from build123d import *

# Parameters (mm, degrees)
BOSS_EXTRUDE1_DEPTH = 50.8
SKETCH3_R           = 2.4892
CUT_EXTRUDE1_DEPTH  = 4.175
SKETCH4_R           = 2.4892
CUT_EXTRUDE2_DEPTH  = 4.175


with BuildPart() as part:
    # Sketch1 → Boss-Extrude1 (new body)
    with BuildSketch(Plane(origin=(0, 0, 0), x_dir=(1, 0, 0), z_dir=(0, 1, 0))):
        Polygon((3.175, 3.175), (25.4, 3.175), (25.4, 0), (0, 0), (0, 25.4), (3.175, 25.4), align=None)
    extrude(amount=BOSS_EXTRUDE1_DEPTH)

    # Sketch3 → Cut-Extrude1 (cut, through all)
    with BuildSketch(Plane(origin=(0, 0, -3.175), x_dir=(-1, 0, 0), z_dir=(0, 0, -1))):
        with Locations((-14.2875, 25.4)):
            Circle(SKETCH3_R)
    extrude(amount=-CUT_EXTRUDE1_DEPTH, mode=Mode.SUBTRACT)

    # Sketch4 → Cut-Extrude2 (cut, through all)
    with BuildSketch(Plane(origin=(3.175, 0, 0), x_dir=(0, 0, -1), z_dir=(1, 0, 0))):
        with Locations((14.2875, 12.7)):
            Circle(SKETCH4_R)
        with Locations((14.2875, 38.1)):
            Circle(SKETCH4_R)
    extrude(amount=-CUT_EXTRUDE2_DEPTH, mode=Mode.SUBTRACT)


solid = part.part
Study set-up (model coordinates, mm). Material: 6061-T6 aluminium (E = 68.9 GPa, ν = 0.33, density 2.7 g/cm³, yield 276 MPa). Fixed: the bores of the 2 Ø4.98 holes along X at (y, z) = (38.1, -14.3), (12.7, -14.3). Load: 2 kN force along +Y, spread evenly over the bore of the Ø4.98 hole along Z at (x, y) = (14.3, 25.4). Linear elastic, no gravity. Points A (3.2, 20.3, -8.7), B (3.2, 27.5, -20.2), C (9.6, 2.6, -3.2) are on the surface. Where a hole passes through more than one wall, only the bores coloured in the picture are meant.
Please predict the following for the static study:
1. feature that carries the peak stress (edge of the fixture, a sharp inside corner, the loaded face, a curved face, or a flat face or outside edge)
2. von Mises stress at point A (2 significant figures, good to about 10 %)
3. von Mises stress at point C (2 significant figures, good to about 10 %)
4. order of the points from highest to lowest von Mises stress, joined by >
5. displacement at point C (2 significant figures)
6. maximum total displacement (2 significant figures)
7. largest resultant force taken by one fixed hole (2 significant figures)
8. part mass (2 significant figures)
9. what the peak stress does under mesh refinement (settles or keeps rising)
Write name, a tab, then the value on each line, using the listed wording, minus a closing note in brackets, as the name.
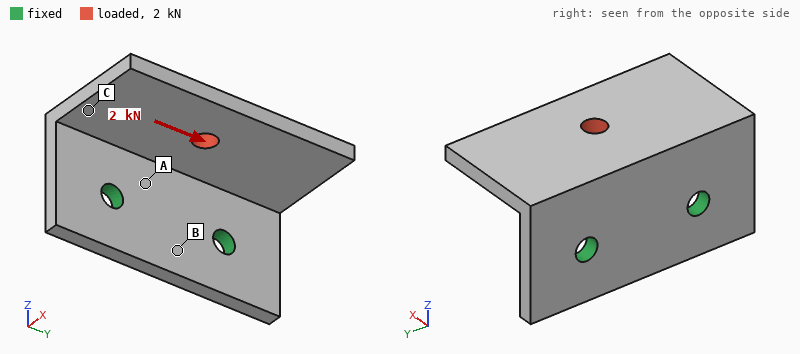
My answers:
feature that carries the peak stress	edge of the fixture
von Mises stress at point A	93 MPa
von Mises stress at point C	51 MPa
order of the points from highest to lowest von Mises stress, joined by >	A > C > B
displacement at point C	0.13 mm
maximum total displacement	0.22 mm
largest resultant force taken by one fixed hole	1.5 kN
part mass	20 g
what the peak stress does under mesh refinement	keeps rising
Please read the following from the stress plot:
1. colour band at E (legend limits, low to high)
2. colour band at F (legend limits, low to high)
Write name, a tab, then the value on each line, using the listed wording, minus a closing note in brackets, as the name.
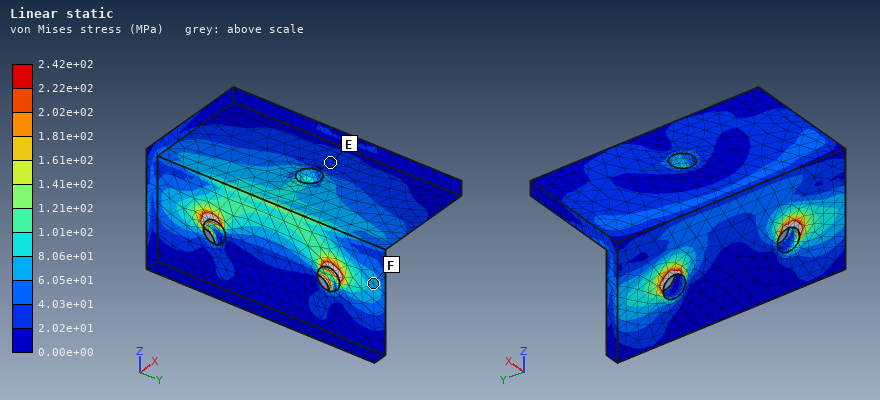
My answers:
colour band at E	2.02e+01 to 4.03e+01 MPa
colour band at F	6.05e+01 to 8.06e+01 MPa
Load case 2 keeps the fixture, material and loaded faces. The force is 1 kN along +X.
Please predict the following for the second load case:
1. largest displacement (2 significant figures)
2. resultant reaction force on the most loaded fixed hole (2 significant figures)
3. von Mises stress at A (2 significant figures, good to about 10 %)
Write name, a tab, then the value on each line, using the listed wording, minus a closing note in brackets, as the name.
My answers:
largest displacement	0.21 mm
resultant reaction force on the most loaded fixed hole	500 N
von Mises stress at A	65 MPa
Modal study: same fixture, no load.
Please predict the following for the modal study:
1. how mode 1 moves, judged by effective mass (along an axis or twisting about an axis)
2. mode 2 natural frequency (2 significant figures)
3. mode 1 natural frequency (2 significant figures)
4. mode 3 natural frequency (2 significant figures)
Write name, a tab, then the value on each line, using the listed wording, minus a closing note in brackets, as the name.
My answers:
how mode 1 moves, judged by effective mass	along Z
mode 2 natural frequency	4300 Hz
mode 1 natural frequency	2600 Hz
mode 3 natural frequency	7000 Hz
